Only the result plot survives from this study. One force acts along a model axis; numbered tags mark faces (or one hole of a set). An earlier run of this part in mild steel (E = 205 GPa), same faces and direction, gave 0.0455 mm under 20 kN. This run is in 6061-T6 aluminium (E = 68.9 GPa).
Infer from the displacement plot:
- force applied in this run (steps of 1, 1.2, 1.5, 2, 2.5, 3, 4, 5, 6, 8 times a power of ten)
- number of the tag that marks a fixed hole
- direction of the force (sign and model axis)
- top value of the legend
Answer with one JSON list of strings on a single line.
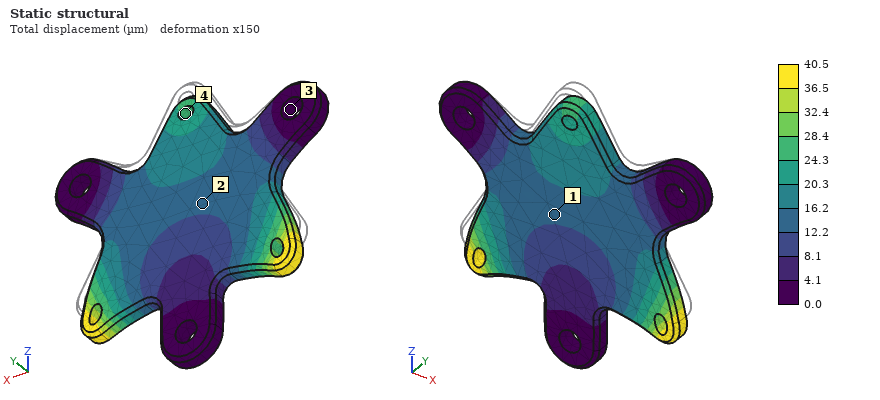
["6 kN", "3", "-Z", "40.5 µm"]
